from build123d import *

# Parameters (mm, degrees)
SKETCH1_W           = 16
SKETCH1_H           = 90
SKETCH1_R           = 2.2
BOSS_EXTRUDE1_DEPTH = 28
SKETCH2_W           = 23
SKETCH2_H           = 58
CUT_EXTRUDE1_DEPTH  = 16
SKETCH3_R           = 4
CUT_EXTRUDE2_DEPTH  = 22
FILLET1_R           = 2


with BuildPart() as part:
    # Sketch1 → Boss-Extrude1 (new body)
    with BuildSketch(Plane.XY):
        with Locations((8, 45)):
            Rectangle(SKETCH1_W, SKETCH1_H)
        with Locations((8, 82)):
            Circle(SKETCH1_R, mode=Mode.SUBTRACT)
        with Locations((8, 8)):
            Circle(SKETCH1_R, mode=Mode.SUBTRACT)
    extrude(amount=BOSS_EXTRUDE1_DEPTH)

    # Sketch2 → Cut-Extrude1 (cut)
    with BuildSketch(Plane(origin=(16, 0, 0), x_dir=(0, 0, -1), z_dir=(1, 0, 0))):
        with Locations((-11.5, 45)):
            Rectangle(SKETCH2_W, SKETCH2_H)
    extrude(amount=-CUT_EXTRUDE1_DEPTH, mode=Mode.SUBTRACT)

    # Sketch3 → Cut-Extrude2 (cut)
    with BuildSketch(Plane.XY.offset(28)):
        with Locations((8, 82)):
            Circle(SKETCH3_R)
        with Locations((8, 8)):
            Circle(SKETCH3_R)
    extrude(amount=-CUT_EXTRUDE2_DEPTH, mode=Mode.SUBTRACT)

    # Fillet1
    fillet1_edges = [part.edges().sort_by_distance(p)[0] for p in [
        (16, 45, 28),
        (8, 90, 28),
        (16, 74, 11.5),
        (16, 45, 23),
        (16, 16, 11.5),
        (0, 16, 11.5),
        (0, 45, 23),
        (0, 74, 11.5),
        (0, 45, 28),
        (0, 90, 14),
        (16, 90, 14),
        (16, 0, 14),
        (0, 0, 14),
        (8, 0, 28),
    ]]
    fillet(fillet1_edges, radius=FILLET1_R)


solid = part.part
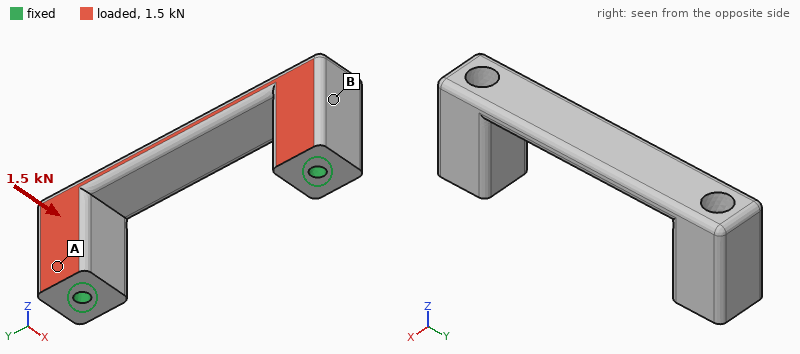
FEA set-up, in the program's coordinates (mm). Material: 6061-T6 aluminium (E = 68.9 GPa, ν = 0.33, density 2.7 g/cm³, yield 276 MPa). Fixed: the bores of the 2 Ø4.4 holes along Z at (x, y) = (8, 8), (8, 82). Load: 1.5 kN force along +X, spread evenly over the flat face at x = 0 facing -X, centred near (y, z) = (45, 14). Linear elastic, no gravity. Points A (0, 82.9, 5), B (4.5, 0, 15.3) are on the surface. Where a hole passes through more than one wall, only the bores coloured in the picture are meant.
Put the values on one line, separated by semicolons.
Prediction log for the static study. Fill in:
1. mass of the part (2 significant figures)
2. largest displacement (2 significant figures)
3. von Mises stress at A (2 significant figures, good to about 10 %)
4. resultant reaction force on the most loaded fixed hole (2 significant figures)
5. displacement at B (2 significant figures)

44 g; 29 µm; 15 MPa; 750 N; 12 µm
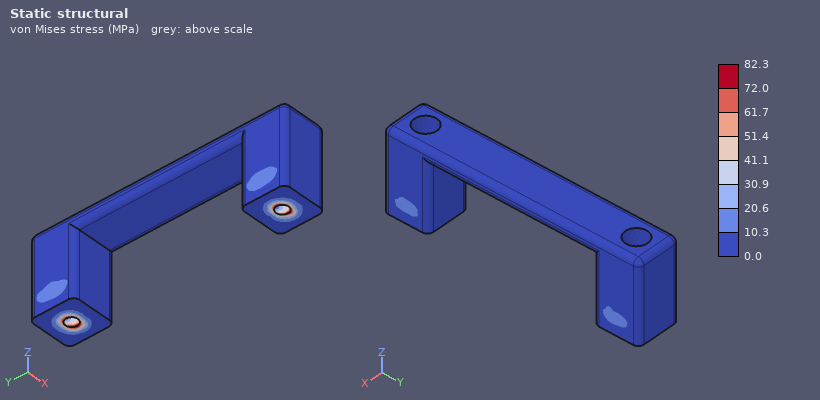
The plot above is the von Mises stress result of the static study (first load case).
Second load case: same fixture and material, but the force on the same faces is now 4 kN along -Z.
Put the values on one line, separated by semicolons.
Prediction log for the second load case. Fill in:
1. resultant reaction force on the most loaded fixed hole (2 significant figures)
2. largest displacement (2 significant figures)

2.0 kN; 72 µm
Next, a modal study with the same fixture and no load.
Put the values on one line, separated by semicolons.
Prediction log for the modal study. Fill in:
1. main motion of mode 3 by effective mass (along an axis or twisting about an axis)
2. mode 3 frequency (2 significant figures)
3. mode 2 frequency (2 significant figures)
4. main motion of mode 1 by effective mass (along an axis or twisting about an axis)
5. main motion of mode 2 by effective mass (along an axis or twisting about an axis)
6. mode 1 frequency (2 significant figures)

along Y; 6100 Hz; 5800 Hz; along X; along Z; 5300 Hz
